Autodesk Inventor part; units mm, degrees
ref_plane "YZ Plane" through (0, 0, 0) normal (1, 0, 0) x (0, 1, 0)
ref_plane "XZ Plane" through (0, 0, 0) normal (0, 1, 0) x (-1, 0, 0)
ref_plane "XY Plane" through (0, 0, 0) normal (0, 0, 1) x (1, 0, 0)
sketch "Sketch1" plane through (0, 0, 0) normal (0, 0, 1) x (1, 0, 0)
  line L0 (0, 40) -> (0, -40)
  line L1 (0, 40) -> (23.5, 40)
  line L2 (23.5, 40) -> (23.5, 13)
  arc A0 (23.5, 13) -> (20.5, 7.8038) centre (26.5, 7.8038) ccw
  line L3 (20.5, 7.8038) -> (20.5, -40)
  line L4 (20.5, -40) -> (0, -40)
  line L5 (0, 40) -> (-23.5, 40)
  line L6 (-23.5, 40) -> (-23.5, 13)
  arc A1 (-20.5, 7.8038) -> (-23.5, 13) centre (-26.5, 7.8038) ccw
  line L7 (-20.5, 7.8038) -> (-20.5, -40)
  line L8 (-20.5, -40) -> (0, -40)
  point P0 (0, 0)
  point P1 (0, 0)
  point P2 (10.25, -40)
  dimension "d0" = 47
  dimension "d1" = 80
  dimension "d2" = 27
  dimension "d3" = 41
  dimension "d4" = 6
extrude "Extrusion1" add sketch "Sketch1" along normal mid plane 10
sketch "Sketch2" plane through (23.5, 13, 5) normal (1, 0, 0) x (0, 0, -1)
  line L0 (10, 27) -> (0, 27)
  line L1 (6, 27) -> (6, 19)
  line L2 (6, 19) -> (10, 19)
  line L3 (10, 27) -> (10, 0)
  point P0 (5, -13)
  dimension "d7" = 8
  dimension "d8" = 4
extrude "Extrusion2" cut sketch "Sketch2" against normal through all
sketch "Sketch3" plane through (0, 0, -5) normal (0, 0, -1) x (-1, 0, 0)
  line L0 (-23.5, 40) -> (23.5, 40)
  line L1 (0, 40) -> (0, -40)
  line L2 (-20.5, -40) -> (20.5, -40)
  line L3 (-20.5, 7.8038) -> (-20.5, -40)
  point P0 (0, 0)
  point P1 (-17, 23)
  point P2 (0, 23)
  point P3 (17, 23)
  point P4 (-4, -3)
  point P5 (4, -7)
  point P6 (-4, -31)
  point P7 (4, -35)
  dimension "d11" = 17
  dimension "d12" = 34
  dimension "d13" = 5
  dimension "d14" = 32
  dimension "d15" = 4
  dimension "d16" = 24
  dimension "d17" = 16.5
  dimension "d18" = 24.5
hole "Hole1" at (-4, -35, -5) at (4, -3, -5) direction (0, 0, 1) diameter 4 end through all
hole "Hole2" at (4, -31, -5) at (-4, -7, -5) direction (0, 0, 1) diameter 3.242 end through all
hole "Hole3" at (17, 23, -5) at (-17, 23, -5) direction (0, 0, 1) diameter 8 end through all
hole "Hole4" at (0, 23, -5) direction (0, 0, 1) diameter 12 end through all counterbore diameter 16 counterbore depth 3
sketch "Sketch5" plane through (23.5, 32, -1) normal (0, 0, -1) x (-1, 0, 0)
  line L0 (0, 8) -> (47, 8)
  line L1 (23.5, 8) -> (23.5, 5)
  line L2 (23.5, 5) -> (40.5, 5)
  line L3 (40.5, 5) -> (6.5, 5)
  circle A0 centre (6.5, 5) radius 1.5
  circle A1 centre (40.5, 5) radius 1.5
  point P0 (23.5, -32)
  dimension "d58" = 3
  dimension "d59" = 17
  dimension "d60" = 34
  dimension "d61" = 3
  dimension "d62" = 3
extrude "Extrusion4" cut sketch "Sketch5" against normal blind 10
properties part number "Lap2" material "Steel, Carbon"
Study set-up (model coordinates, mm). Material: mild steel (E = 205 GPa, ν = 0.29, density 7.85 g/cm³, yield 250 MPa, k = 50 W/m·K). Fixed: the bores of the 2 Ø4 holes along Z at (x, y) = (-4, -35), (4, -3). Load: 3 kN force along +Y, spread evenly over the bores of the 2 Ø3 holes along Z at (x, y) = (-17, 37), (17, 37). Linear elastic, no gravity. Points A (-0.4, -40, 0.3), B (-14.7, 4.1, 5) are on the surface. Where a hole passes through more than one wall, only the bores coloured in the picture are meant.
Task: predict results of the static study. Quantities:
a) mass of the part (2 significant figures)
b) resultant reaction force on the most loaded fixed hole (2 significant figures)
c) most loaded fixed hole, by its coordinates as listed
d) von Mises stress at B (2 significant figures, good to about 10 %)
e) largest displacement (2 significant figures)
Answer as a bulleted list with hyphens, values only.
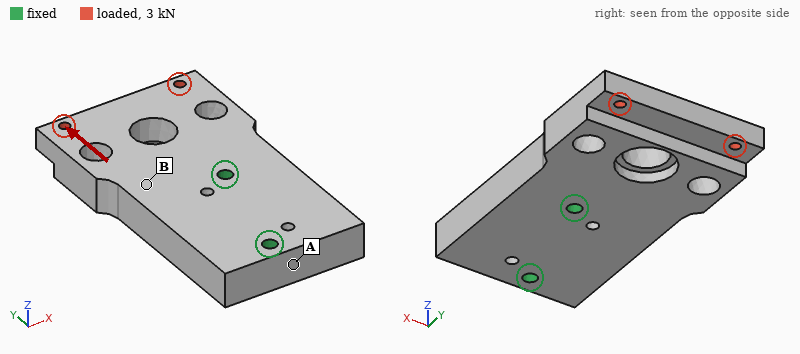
- 240 g
- 2.2 kN
- (4, -3)
- 14 MPa
- 13 µm
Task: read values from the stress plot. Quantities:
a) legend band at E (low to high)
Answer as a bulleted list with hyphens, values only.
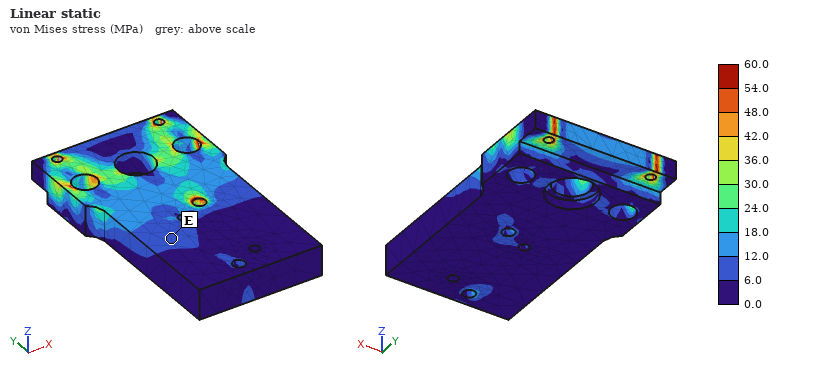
- 6.0 to 12.0 MPa
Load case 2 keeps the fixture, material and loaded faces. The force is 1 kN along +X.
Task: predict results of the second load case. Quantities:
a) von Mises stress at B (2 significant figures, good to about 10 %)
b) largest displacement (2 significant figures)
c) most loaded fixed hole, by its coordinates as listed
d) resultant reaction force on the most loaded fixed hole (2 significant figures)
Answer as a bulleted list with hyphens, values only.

- 8.4 MPa
- 11 µm
- (4, -3)
- 2.1 kN
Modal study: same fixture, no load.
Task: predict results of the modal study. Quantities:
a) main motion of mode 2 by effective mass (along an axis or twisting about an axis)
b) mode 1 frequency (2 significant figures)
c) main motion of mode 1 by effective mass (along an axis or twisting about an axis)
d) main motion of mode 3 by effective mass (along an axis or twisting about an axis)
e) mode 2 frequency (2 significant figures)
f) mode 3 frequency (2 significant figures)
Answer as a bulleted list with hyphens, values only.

- twisting about Y
- 4000 Hz
- along Z
- along X
- 6200 Hz
- 8200 Hz
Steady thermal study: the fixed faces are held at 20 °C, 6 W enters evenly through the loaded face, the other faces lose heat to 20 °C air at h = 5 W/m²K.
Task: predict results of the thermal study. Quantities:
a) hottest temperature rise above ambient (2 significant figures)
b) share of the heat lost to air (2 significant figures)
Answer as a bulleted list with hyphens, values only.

- 21 K
- 5.1 %
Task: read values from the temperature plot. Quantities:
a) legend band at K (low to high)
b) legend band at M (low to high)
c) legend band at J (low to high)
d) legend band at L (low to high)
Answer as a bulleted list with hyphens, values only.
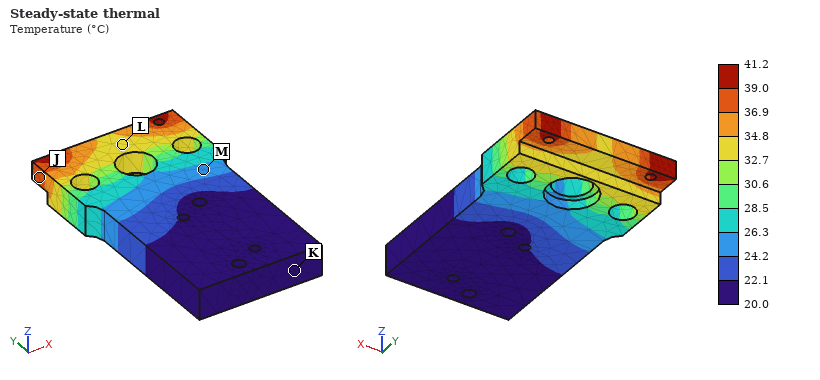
- 20.0 to 22.1 °C
- 24.2 to 26.3 °C
- 36.9 to 39.0 °C
- 32.7 to 34.8 °C
